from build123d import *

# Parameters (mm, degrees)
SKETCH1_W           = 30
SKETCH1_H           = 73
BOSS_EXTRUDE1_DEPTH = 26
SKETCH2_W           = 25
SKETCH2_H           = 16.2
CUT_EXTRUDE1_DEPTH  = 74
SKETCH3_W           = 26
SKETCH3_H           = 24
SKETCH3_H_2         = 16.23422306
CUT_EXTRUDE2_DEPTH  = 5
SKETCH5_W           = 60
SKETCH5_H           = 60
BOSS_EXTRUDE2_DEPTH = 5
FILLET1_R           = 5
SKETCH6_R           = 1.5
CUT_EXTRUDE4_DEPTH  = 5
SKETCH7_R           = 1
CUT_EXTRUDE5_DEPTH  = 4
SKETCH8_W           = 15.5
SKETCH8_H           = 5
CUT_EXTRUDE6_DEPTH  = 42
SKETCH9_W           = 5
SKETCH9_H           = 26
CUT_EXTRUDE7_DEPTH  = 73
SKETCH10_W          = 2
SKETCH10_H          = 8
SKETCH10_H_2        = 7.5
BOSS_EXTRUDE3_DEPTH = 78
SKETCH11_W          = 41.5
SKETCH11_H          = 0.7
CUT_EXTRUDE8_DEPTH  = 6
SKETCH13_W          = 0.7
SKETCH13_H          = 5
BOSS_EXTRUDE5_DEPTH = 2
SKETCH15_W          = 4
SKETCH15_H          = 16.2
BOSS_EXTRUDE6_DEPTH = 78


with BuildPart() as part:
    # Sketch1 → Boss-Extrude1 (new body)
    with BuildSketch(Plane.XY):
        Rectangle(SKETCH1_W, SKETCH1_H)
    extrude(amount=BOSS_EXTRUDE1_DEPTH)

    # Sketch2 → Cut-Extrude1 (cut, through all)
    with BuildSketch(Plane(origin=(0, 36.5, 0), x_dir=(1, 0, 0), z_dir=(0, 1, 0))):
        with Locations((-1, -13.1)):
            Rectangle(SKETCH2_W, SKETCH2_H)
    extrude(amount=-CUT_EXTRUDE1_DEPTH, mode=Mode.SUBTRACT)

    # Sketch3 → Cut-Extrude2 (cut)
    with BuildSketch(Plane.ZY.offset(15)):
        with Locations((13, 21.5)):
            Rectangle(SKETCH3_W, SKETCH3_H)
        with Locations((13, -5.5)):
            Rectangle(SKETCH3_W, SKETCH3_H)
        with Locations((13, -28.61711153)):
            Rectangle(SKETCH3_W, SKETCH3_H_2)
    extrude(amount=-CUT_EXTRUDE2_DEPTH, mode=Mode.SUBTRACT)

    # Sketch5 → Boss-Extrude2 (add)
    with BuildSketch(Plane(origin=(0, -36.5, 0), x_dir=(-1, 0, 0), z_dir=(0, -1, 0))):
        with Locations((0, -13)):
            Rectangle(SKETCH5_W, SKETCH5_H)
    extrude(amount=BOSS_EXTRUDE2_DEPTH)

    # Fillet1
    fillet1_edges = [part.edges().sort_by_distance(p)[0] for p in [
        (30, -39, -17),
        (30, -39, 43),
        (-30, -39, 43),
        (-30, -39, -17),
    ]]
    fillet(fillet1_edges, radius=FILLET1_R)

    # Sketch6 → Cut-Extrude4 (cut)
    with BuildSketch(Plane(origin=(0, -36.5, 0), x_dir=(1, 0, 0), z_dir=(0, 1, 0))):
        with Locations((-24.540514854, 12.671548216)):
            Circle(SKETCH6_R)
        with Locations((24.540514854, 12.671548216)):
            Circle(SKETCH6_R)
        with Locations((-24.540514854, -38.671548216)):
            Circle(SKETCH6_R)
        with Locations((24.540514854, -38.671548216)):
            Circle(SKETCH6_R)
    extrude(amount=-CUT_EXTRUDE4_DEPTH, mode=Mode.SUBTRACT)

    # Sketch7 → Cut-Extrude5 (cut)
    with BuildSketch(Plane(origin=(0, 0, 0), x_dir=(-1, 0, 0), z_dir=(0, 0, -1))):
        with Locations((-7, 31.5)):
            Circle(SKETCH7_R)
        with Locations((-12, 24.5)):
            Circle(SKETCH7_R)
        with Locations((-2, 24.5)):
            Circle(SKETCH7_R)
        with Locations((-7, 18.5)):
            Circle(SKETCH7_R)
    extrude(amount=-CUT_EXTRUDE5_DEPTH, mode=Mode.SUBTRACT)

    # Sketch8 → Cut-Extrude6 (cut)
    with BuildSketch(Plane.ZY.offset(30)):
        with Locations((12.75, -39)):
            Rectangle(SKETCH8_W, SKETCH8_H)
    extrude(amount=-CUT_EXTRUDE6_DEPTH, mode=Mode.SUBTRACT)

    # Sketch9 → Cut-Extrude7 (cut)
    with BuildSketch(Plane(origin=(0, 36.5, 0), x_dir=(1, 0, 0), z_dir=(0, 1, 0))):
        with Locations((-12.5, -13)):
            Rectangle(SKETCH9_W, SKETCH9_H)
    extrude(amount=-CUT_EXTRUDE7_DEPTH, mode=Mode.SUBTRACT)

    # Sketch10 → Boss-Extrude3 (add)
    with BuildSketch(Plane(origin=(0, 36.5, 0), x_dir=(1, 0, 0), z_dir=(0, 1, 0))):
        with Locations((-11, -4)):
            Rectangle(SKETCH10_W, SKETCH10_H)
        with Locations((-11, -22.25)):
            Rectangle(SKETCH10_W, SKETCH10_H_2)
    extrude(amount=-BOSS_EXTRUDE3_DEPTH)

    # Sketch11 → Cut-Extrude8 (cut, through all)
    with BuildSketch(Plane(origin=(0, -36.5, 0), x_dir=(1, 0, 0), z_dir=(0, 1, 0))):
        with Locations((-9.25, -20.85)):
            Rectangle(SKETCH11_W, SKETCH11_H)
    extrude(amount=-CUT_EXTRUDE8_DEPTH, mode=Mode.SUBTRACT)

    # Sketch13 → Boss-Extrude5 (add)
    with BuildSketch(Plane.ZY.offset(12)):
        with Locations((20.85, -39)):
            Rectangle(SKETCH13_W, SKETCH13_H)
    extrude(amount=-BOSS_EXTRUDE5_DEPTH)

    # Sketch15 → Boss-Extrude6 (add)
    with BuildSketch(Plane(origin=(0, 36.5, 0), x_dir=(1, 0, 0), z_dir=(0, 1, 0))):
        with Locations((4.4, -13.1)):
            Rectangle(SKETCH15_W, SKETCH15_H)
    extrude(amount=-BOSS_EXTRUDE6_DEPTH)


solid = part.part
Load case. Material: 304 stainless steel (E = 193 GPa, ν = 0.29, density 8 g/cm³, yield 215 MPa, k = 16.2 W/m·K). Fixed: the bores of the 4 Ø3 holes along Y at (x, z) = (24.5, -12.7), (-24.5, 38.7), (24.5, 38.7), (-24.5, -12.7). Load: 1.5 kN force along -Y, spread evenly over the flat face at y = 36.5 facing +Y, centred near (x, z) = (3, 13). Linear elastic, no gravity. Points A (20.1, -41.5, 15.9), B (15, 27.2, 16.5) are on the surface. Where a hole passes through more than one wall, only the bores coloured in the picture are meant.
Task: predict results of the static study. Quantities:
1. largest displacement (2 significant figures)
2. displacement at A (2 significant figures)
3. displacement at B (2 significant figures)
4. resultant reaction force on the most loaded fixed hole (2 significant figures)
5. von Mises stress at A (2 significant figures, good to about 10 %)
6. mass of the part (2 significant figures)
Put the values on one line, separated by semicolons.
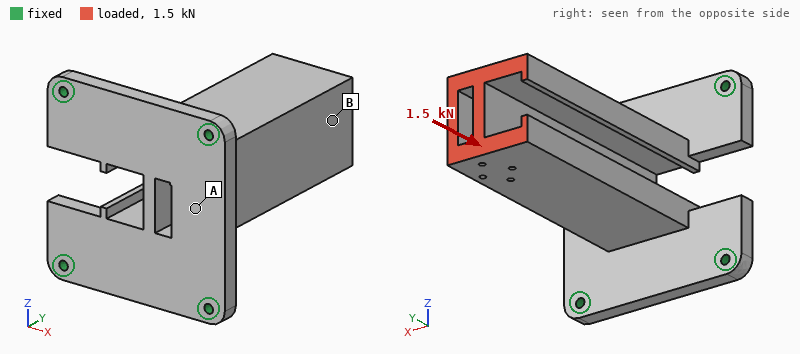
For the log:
16 µm; 9.4 µm; 13 µm; 450 N; 15 MPa; 350 g
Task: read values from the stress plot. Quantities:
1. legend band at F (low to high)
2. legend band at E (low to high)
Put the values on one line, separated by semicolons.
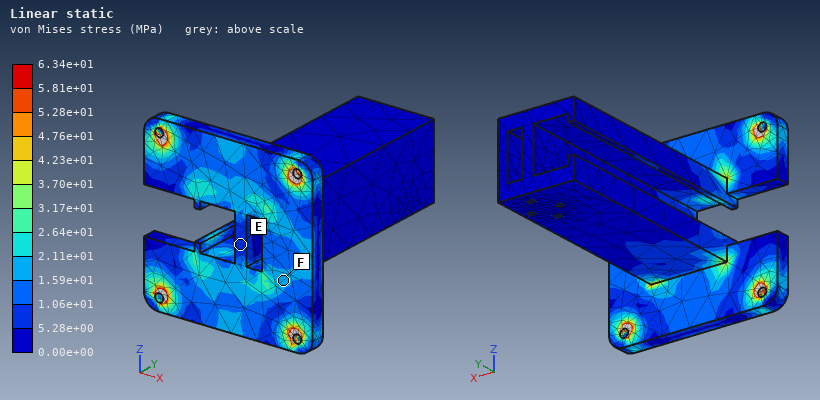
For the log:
1.59e+01 to 2.11e+01 MPa; 5.28e+00 to 1.06e+01 MPa
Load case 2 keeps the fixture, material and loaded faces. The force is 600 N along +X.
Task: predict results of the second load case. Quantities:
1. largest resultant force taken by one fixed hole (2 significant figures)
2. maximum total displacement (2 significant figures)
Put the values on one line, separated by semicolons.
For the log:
570 N; 95 µm
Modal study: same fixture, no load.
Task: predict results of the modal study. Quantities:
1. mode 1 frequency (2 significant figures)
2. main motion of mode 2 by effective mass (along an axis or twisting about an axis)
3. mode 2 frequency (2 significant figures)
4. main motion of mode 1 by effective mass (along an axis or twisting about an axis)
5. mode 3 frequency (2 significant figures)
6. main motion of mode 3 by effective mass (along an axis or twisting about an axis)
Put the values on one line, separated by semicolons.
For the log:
1400 Hz; along Z; 1500 Hz; along X; 3400 Hz; along Y
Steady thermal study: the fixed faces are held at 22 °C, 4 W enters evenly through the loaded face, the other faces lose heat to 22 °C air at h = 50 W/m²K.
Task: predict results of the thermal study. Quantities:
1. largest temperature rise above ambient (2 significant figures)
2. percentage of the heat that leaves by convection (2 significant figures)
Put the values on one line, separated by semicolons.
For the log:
16 K; 96 %
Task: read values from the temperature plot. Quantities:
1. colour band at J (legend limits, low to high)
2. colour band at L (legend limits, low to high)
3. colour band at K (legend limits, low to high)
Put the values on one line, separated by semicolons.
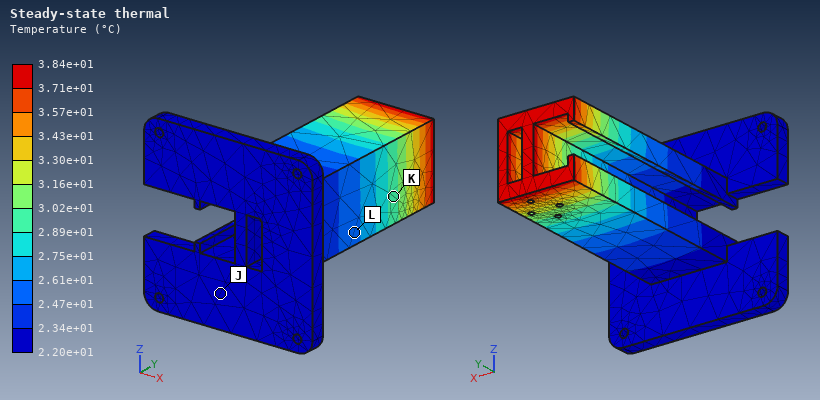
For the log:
2.20e+01 to 2.34e+01 °C; 2.47e+01 to 2.61e+01 °C; 2.89e+01 to 3.02e+01 °C
